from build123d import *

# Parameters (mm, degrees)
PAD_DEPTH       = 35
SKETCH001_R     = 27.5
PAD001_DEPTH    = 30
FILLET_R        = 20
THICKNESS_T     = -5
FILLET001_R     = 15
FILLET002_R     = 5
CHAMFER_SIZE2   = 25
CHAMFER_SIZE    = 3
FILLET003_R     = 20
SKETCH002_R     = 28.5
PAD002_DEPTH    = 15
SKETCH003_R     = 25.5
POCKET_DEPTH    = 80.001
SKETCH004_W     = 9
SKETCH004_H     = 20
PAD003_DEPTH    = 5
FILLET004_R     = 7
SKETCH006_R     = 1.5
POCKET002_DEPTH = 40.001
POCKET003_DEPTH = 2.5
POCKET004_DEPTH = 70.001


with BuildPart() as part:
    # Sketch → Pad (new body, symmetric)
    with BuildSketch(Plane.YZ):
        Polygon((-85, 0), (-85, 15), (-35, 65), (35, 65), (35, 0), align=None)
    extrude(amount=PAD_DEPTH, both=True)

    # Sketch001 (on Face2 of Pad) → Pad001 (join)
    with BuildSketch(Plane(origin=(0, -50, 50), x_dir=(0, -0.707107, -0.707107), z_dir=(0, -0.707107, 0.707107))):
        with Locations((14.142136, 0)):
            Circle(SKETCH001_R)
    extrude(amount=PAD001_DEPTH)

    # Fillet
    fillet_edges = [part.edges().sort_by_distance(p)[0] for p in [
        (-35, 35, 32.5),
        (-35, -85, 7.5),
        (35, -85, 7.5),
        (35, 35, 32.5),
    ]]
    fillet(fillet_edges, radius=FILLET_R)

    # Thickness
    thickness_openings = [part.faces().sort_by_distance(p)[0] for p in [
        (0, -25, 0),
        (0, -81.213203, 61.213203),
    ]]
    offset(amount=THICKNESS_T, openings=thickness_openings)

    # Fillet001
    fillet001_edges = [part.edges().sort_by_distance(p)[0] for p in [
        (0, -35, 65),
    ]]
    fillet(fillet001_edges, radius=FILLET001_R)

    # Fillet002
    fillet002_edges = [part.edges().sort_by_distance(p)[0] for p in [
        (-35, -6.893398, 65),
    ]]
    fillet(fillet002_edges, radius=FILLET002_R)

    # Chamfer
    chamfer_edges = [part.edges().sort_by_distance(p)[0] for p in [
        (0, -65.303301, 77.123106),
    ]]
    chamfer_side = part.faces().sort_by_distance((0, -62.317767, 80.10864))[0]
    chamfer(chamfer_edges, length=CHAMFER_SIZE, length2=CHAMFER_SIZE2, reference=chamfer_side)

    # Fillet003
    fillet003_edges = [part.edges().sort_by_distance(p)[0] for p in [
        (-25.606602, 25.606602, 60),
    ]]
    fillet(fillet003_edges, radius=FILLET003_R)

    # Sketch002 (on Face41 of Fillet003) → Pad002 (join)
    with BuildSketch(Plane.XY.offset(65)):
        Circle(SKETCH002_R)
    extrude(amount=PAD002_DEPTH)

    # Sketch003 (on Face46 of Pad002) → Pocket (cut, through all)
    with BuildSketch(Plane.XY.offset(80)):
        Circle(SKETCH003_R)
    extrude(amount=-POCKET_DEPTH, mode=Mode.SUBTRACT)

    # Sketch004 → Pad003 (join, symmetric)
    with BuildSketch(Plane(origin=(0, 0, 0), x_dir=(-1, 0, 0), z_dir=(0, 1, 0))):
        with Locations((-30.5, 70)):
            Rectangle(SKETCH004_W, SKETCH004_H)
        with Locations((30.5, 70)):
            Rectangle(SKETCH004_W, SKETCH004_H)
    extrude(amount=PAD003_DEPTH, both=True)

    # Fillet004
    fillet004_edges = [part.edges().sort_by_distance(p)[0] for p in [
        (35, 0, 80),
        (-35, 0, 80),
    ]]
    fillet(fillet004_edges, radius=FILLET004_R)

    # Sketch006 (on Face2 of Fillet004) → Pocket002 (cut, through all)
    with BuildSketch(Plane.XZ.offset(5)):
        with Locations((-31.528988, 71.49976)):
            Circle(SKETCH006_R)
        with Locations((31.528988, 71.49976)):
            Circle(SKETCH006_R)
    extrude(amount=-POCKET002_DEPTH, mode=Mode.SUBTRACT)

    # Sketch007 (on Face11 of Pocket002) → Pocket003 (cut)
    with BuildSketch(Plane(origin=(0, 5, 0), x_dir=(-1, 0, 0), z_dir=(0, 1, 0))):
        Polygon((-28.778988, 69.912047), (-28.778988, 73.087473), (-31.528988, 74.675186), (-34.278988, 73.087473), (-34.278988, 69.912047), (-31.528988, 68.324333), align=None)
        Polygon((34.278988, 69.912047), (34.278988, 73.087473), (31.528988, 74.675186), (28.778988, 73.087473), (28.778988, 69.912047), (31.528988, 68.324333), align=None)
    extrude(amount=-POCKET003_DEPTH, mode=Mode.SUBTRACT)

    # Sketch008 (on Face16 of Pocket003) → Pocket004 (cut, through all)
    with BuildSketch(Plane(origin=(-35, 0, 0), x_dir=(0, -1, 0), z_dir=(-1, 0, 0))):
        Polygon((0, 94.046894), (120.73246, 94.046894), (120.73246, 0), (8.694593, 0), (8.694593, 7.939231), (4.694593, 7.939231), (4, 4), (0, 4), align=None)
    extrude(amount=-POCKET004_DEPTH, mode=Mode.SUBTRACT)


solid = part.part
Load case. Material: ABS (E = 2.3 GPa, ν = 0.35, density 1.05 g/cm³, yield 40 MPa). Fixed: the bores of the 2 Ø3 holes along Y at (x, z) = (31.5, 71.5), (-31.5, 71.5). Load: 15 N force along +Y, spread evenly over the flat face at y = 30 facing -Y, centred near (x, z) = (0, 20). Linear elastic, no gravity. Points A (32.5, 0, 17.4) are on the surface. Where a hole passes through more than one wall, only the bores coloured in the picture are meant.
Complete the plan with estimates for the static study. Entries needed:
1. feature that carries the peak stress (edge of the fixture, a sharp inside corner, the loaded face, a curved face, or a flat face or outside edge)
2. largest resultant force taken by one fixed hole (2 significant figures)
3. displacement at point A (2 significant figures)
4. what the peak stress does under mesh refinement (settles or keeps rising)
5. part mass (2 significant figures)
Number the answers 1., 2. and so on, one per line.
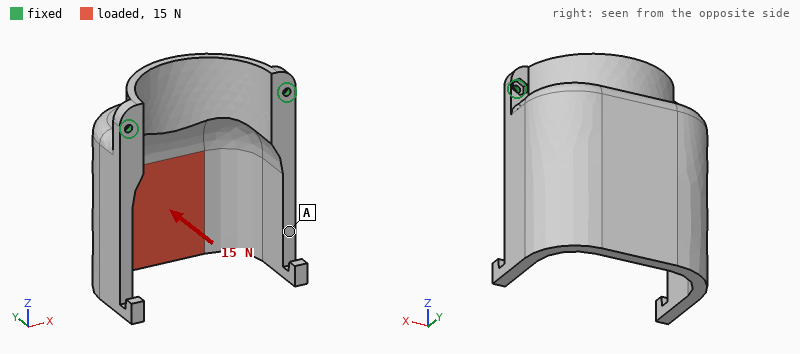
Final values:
1. edge of the fixture
2. 7.5 N
3. 0.70 mm
4. keeps rising
5. 54 g
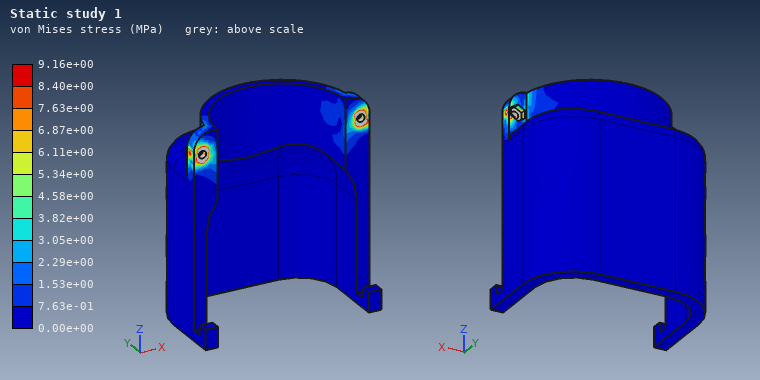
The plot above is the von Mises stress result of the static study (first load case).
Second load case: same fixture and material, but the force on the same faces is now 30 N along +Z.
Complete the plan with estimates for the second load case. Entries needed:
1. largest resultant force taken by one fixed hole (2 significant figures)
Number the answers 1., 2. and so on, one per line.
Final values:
1. 15 N
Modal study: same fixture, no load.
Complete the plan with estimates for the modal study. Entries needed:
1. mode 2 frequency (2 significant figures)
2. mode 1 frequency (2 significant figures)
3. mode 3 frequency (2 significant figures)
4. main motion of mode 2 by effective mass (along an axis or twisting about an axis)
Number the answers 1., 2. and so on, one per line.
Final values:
1. 350 Hz
2. 120 Hz
3. 850 Hz
4. along X
